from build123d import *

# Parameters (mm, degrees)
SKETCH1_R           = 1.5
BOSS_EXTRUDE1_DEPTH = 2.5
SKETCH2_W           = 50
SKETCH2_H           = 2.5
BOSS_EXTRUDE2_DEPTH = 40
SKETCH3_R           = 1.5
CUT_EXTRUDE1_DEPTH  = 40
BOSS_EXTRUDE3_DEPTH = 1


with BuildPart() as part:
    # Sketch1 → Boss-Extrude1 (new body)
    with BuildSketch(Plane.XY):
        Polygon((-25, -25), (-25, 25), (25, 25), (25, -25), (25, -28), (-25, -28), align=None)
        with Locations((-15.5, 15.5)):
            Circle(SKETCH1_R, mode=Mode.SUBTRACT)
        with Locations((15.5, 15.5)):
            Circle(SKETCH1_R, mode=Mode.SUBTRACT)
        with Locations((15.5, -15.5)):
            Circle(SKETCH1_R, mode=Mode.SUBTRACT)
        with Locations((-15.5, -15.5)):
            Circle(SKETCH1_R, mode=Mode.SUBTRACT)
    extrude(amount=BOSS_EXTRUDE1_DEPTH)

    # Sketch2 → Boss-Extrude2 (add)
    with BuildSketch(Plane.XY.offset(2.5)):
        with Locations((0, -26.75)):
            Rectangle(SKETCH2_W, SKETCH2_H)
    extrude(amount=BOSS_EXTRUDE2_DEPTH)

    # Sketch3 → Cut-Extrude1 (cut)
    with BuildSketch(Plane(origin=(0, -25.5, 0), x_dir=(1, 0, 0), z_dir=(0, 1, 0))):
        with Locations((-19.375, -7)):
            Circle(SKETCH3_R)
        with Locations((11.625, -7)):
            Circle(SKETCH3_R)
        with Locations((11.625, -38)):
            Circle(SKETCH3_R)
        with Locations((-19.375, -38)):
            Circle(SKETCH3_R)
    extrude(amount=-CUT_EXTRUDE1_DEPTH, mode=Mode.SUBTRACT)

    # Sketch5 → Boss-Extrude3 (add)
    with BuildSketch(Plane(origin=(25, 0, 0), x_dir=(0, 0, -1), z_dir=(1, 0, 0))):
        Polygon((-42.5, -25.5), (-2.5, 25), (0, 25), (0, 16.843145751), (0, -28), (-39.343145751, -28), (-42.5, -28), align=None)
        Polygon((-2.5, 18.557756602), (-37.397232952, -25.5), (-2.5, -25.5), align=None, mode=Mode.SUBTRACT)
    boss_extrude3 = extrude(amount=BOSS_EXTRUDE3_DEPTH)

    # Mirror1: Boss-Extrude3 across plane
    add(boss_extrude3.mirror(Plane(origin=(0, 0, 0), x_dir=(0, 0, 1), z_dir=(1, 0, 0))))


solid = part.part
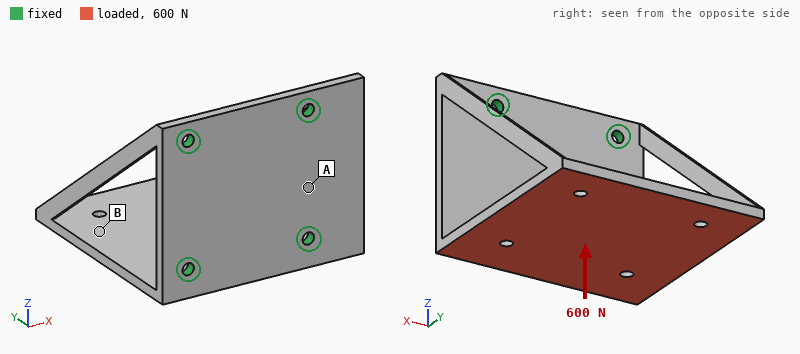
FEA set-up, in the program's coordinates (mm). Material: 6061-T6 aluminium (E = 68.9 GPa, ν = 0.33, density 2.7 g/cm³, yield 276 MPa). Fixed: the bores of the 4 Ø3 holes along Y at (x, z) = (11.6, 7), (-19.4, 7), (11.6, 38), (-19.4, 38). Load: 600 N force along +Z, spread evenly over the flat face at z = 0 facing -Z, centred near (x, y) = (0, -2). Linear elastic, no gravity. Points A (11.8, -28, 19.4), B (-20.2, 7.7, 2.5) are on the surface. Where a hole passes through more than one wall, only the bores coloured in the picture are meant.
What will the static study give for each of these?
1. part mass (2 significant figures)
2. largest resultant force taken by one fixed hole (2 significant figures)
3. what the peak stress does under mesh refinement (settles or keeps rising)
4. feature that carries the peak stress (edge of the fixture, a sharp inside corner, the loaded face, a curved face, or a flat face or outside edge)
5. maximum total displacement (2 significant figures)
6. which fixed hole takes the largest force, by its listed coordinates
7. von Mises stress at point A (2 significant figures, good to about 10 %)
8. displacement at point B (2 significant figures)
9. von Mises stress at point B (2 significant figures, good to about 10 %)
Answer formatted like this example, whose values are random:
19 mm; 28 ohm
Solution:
34 g; 310 N; keeps rising; edge of the fixture; 0.36 mm; (11.6, 7); 18 MPa; 0.20 mm; 55 MPa
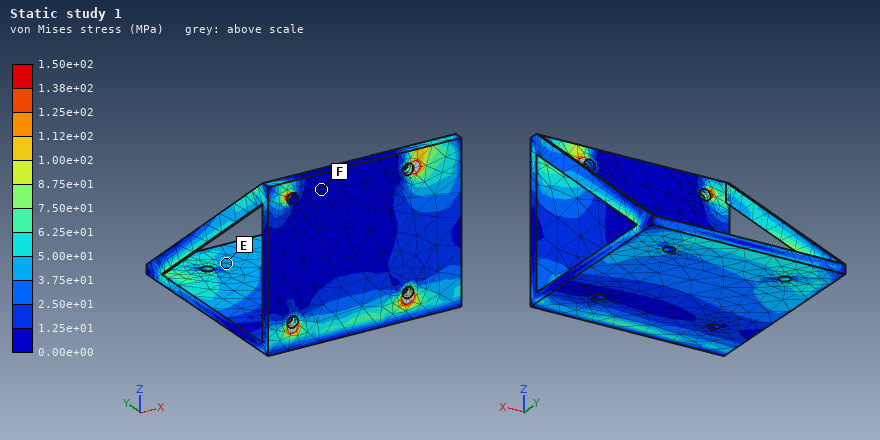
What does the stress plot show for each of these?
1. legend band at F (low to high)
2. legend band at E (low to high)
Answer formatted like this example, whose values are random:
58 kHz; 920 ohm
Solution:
0.00e+00 to 1.25e+01 MPa; 3.75e+01 to 5.00e+01 MPa
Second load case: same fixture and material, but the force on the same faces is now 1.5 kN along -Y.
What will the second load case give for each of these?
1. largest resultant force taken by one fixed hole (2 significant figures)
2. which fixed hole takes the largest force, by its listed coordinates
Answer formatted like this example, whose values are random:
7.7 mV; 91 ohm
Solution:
1.0 kN; (11.6, 7)
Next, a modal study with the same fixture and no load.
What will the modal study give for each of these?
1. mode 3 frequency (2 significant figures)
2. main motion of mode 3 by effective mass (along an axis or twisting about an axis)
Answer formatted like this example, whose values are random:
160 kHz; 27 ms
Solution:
1800 Hz; along Z
